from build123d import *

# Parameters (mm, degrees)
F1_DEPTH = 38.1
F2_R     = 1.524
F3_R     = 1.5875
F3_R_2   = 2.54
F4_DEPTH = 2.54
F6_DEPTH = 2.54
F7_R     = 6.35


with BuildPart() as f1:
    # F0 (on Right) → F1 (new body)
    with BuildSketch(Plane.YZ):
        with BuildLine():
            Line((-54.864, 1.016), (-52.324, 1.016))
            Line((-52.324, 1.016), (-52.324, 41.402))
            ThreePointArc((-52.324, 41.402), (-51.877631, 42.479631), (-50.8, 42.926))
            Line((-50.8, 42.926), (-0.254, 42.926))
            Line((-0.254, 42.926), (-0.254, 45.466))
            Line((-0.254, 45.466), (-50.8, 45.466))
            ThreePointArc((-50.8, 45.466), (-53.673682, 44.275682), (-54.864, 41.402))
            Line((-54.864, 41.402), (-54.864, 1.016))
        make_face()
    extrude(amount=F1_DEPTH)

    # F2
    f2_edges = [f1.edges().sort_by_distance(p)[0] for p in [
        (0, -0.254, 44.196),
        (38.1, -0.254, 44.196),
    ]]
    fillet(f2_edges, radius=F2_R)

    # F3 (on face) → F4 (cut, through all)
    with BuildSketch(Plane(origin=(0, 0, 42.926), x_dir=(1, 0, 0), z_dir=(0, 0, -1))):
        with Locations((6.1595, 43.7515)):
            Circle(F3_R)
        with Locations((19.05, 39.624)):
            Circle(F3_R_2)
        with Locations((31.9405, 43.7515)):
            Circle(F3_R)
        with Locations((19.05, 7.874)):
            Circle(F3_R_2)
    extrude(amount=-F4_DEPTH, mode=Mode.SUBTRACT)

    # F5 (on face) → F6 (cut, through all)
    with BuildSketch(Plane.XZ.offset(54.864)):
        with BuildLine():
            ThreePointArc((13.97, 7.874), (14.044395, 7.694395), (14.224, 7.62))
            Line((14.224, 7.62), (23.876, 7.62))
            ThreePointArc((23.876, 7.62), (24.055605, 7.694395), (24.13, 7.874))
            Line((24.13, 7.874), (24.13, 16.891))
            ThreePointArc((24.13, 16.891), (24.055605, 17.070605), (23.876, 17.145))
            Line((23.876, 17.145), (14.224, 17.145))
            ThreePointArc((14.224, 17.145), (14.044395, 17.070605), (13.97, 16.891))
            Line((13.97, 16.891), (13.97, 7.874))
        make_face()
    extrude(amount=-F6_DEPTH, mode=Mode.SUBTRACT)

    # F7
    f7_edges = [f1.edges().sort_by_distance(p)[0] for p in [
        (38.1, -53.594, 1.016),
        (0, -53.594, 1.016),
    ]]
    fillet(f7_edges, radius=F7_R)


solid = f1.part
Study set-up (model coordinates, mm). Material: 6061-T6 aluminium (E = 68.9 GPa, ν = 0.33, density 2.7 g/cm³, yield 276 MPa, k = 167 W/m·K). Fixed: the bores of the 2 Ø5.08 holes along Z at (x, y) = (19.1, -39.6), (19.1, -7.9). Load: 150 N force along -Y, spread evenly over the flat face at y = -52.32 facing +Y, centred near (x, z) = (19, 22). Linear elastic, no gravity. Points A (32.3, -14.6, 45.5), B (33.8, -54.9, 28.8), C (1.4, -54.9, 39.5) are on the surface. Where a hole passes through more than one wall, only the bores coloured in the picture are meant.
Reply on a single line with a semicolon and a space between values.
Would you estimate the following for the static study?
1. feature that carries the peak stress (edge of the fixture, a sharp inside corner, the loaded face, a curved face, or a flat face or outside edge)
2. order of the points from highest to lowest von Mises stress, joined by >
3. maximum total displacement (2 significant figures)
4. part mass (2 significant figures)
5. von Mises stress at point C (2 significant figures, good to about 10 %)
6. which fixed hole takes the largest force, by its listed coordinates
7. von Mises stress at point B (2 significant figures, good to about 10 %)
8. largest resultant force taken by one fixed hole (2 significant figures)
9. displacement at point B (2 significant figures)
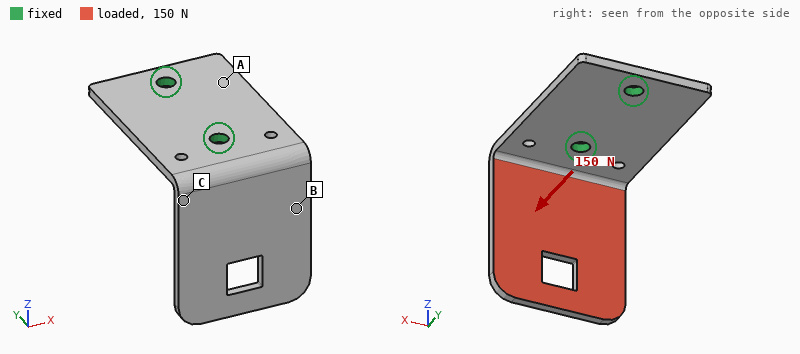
a flat face or outside edge; C > B > A; 0.94 mm; 24 g; 62 MPa; (19.1, -39.6); 32 MPa; 130 N; 0.29 mm
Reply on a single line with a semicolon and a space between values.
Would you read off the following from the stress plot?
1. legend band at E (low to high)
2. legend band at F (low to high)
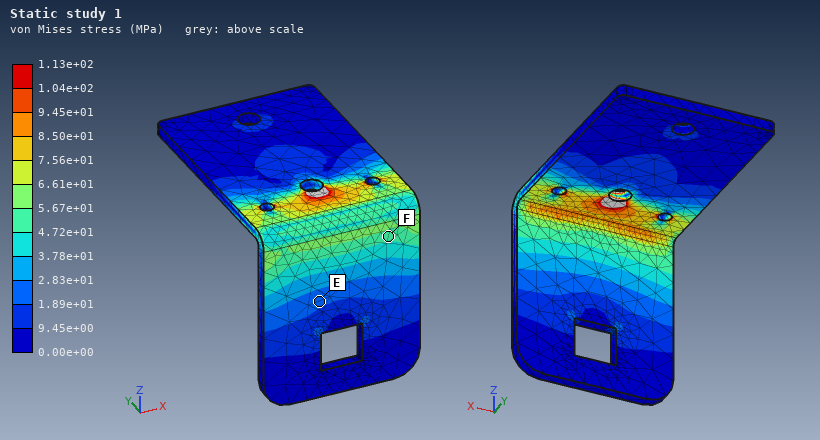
1.89e+01 to 2.83e+01 MPa; 4.72e+01 to 5.67e+01 MPa
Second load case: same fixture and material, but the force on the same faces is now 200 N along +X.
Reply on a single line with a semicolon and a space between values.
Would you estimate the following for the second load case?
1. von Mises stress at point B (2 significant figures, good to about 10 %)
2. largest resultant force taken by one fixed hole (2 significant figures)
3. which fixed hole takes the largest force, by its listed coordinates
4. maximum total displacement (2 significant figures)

14 MPa; 260 N; (19.1, -39.6); 0.44 mm
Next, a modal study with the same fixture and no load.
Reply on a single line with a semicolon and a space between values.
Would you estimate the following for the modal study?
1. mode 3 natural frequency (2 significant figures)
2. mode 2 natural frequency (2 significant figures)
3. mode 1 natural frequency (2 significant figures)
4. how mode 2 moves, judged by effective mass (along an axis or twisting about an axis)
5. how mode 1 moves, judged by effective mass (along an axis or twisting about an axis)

2800 Hz; 1200 Hz; 790 Hz; along X; along Y
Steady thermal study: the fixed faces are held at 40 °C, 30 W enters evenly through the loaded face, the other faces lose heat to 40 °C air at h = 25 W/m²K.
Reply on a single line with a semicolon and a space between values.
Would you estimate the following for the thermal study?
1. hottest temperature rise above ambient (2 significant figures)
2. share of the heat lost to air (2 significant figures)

69 K; 12 %
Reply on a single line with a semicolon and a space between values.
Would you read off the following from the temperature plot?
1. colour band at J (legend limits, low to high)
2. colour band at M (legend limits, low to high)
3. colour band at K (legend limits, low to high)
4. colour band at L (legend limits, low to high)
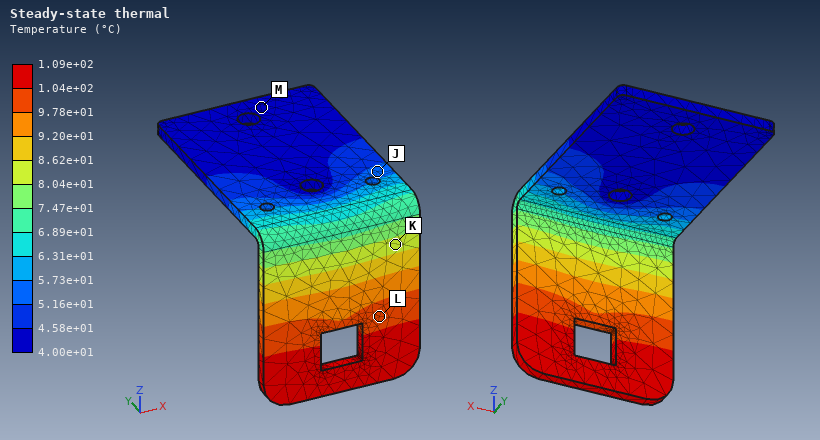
5.16e+01 to 5.73e+01 °C; 4.00e+01 to 4.58e+01 °C; 8.04e+01 to 8.62e+01 °C; 9.78e+01 to 1.04e+02 °C
